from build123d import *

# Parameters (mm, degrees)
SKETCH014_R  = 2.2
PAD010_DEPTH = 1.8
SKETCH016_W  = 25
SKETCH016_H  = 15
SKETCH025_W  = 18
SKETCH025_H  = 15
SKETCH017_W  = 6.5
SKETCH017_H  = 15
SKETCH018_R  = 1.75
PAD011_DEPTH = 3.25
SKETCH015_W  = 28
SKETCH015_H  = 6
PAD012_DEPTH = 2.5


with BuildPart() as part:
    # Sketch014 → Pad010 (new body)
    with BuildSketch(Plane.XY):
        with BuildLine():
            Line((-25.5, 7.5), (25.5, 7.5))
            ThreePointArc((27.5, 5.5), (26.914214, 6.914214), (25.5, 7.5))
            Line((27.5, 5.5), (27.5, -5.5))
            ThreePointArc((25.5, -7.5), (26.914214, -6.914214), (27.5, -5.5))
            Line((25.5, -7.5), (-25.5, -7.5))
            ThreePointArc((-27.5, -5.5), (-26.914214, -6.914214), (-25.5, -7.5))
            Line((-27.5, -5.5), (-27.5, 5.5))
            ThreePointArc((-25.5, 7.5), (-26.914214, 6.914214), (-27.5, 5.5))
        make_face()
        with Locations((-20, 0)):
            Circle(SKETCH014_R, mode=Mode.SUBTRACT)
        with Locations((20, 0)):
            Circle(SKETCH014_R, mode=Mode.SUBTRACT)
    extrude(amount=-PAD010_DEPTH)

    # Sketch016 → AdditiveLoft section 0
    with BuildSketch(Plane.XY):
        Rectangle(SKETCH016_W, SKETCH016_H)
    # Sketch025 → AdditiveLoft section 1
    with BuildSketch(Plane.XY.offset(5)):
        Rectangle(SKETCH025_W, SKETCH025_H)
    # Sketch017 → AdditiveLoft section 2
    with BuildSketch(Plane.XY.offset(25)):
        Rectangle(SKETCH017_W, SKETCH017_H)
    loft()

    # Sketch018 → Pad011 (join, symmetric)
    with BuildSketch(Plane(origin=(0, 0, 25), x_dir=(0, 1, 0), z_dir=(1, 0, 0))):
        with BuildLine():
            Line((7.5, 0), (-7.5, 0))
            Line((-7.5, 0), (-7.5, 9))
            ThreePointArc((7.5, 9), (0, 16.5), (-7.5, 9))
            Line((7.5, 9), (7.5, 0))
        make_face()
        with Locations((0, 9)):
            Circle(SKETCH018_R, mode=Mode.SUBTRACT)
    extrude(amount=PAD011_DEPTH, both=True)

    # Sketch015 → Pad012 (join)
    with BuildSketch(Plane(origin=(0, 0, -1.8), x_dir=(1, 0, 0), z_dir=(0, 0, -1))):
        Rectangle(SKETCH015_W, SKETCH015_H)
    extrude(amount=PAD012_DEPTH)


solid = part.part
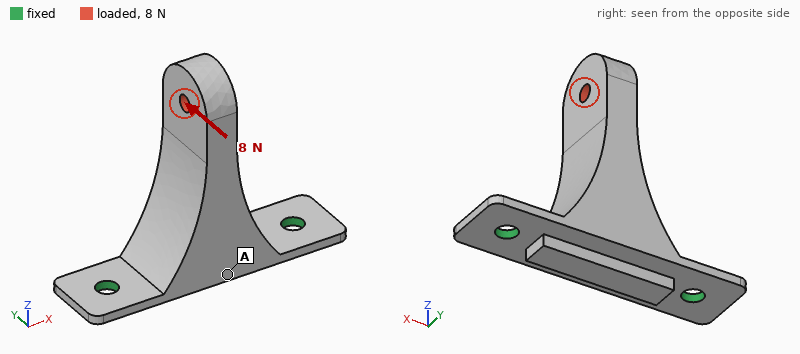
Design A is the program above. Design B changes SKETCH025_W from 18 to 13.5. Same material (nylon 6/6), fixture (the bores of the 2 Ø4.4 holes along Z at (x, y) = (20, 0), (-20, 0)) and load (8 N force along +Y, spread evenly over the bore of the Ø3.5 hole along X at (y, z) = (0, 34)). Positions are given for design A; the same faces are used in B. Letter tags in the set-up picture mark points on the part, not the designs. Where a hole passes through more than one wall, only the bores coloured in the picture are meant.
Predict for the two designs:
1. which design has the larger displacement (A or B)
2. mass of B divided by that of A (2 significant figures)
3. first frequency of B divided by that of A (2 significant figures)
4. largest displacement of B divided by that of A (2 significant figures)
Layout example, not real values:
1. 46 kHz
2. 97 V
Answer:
1. B
2. 0.84
3. 1.0
4. 1.1
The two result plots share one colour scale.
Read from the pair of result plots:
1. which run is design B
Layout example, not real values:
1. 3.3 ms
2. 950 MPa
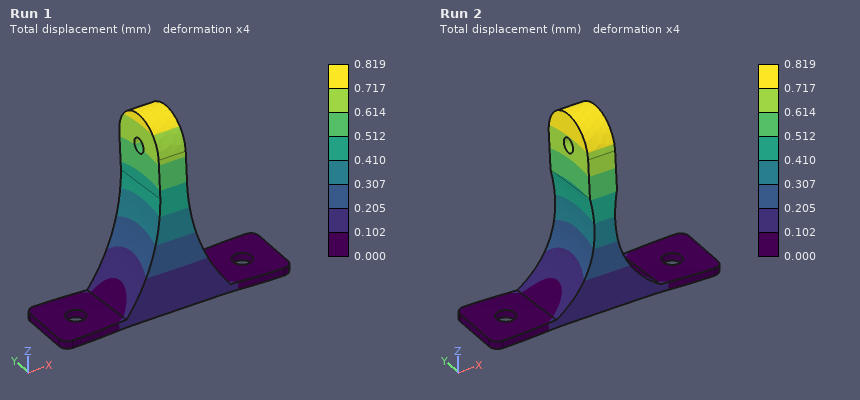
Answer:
1. Run 2
